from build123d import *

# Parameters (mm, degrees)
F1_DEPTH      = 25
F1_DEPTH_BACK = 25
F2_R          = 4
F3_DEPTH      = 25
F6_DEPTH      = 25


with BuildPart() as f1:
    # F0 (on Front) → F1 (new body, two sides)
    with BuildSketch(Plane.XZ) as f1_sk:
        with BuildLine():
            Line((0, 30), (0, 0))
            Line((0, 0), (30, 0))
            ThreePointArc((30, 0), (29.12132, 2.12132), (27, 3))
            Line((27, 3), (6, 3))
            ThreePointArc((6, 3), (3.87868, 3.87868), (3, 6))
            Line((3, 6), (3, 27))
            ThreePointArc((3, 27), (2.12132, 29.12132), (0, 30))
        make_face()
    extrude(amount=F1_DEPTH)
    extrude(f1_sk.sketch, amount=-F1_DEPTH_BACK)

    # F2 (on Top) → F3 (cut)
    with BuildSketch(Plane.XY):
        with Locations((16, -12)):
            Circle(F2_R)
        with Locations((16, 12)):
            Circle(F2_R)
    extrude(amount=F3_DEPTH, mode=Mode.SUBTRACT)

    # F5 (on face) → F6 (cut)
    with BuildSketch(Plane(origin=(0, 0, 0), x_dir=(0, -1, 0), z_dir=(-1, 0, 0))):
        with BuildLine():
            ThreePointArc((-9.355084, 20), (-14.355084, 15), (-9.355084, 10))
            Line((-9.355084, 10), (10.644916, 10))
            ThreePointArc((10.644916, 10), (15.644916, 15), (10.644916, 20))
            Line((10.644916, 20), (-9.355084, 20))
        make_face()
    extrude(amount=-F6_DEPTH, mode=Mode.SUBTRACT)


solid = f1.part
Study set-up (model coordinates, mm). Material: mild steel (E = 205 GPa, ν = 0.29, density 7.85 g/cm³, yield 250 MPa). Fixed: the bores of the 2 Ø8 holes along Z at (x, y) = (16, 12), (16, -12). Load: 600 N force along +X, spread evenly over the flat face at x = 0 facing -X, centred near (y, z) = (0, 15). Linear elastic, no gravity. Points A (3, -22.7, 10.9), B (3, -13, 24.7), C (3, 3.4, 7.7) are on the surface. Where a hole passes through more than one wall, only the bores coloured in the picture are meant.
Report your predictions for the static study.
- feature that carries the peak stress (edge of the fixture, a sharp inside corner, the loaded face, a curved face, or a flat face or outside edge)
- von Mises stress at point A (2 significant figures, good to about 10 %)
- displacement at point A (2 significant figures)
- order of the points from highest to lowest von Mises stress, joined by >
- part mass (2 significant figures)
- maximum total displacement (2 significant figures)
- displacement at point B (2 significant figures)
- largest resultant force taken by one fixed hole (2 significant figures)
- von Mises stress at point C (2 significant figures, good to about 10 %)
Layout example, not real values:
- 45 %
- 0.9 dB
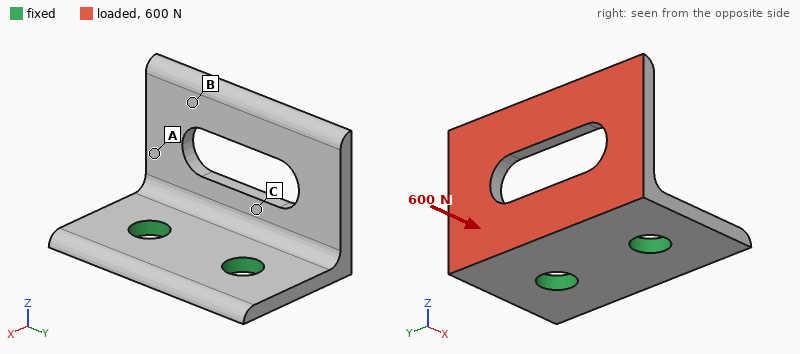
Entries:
- a flat face or outside edge
- 110 MPa
- 0.048 mm
- A > C > B
- 57 g
- 0.22 mm
- 0.16 mm
- 300 N
- 31 MPa
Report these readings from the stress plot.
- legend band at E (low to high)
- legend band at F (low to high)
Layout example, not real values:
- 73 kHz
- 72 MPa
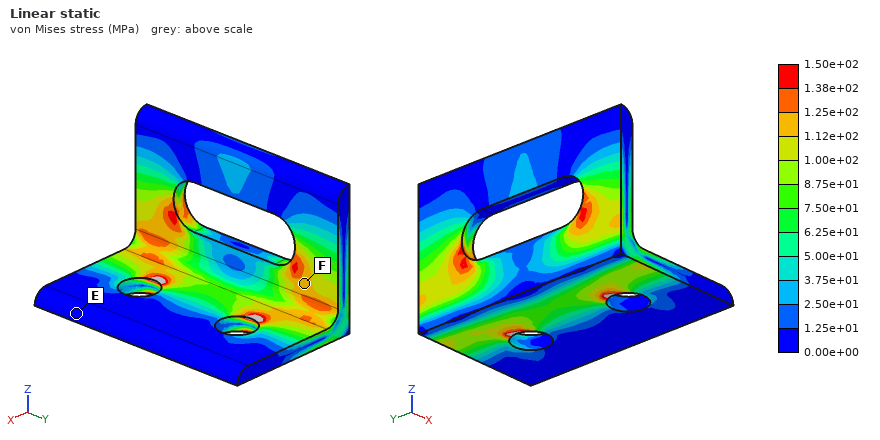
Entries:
- 0.00e+00 to 1.25e+01 MPa
- 1.12e+02 to 1.25e+02 MPa
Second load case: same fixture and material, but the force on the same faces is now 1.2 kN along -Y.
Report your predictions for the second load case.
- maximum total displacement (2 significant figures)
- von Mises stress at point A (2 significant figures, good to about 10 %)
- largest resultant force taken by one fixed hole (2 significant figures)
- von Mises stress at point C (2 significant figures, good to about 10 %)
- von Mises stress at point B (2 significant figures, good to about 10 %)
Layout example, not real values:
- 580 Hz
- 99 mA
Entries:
- 55 µm
- 44 MPa
- 980 N
- 51 MPa
- 12 MPa
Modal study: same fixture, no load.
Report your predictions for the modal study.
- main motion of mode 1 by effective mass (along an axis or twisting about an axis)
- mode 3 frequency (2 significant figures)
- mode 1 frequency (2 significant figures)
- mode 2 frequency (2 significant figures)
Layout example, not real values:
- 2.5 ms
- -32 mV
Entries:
- along X
- 5600 Hz
- 1900 Hz
- 3500 Hz
